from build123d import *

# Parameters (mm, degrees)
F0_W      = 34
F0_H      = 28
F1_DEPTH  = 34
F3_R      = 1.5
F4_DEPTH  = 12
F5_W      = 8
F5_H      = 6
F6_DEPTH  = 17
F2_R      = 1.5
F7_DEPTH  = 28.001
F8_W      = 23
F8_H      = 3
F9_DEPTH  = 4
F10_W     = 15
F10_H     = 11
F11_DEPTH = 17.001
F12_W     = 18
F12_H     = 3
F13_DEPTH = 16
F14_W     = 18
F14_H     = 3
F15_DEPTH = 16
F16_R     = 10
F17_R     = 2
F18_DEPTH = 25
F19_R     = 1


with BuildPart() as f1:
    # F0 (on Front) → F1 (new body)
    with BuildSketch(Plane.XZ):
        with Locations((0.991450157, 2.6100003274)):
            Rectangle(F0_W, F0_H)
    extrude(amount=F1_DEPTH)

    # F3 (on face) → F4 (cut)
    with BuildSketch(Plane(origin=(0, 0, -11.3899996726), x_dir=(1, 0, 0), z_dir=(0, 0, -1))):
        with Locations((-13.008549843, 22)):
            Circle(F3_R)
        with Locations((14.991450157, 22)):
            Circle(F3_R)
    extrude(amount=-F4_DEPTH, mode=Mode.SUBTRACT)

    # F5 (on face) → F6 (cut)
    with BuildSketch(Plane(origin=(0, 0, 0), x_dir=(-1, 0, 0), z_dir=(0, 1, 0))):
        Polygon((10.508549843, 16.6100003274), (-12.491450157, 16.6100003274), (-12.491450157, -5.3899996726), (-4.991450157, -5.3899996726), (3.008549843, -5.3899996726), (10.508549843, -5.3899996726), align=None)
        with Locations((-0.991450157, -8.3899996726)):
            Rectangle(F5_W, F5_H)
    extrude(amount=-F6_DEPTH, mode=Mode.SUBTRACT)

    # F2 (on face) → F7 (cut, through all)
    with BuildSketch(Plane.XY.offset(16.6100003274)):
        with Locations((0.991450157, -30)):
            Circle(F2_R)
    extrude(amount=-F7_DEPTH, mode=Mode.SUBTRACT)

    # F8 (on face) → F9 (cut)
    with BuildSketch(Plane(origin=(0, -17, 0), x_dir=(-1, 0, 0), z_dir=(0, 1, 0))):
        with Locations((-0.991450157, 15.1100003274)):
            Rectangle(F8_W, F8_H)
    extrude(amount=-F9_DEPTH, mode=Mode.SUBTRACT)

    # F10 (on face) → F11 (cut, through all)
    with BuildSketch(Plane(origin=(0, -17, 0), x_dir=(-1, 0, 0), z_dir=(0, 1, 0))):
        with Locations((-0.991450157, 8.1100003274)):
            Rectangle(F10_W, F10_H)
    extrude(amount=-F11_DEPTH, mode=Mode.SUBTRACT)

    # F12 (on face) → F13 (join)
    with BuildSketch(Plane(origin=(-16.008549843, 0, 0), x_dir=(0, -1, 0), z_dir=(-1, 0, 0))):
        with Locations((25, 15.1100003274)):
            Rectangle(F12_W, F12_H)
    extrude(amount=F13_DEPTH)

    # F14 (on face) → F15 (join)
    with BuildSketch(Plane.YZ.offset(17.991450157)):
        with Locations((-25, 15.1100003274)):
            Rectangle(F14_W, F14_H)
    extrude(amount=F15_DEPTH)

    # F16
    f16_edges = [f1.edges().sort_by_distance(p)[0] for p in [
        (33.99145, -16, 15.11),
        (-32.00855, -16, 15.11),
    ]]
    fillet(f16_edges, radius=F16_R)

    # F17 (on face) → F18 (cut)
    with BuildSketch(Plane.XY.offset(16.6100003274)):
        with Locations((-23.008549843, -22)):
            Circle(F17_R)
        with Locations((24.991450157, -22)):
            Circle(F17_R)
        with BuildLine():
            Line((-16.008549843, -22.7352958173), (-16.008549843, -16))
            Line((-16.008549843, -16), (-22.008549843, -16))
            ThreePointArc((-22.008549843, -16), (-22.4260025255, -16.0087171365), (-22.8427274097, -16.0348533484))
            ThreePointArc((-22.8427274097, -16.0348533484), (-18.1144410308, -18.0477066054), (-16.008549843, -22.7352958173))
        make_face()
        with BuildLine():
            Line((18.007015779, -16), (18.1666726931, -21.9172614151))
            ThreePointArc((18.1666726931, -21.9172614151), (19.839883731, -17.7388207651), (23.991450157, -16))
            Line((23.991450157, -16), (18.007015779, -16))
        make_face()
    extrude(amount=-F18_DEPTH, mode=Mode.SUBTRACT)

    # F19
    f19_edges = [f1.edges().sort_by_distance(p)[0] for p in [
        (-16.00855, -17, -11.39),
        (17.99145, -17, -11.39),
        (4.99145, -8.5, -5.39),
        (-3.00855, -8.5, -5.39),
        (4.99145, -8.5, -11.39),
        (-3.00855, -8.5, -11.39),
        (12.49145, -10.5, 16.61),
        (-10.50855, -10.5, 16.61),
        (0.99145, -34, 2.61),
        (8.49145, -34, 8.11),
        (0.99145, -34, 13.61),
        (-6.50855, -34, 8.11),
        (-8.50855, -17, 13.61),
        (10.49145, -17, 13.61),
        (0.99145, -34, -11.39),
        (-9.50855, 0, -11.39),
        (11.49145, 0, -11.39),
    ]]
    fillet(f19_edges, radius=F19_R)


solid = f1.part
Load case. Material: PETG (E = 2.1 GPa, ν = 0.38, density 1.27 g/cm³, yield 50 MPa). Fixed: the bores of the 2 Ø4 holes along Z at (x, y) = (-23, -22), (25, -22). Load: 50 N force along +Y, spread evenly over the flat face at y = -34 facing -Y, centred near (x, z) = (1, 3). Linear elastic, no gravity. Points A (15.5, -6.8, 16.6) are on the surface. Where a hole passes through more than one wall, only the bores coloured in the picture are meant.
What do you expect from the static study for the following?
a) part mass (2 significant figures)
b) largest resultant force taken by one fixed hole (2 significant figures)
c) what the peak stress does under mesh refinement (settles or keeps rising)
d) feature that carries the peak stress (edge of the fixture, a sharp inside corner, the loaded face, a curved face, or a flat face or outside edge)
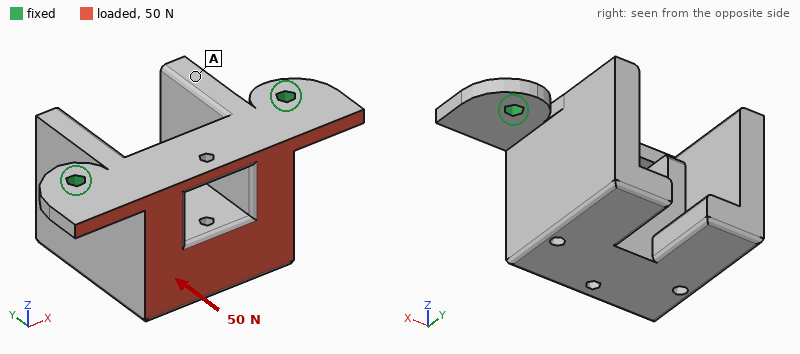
27 g
30 N
keeps rising
a sharp inside corner
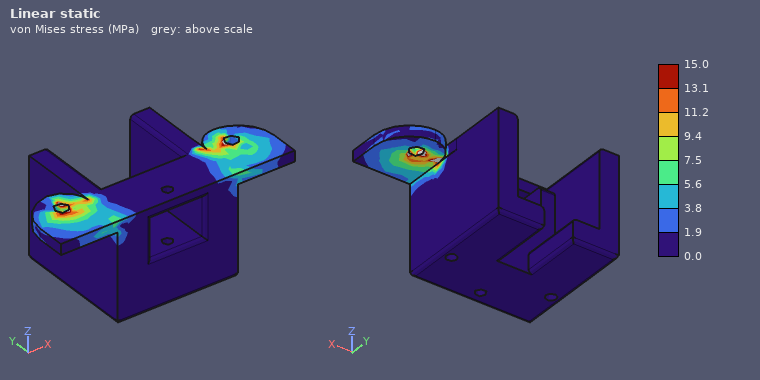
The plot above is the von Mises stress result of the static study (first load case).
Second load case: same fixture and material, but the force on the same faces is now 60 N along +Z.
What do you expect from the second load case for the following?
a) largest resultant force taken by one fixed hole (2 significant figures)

31 N
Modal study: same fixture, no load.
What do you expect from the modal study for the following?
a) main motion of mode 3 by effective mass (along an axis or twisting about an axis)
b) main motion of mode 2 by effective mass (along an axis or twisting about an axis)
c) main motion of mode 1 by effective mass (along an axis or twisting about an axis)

along Z
along X
along Y
